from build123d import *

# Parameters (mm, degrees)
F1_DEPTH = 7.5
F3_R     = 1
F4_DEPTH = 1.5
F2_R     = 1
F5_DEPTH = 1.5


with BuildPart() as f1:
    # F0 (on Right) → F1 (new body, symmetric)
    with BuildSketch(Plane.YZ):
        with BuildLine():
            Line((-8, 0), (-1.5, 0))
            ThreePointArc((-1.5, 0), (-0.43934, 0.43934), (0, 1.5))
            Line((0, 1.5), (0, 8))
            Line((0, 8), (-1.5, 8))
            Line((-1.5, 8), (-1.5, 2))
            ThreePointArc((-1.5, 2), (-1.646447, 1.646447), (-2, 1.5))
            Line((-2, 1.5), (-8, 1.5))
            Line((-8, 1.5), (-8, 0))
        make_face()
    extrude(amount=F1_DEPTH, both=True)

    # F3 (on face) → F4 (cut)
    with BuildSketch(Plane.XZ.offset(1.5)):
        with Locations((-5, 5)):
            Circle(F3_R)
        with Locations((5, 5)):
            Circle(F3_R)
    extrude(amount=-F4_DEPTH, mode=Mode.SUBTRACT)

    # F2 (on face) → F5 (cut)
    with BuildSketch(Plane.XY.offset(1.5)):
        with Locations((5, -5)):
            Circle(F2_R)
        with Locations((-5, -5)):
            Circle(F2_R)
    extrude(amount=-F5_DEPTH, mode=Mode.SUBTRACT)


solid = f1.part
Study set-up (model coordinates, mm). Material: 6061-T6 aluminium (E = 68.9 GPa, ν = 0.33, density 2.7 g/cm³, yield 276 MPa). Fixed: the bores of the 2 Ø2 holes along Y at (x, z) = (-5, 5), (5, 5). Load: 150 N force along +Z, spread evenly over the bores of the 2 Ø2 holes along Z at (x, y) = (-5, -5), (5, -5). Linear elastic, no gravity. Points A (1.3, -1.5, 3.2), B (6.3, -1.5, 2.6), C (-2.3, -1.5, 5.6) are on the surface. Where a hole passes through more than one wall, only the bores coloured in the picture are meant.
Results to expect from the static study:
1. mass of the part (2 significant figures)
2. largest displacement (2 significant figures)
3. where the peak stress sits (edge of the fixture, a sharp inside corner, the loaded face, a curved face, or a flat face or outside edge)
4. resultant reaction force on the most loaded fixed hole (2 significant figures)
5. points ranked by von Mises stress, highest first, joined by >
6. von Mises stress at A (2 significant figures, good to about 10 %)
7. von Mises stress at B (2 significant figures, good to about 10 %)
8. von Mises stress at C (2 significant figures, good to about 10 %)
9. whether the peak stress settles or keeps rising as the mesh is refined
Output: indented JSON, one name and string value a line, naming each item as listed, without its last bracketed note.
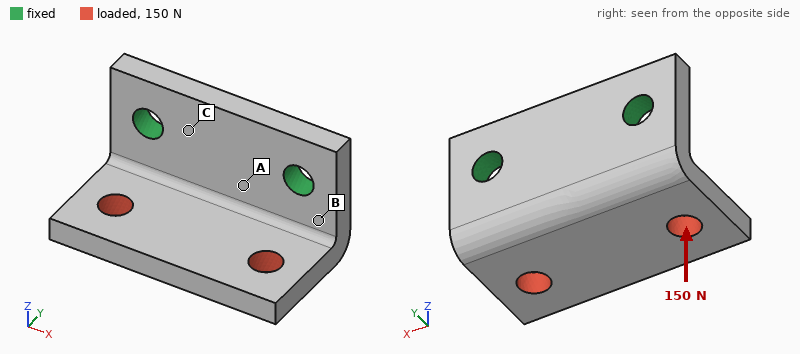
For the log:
{
  "mass of the part": "0.81 g",
  "largest displacement": "82 µm",
  "where the peak stress sits": "edge of the fixture",
  "resultant reaction force on the most loaded fixed hole": "76 N",
  "points ranked by von Mises stress, highest first, joined by >": "B > A > C",
  "von Mises stress at A": "78 MPa",
  "von Mises stress at B": "120 MPa",
  "von Mises stress at C": "32 MPa",
  "whether the peak stress settles or keeps rising as the mesh is refined": "keeps rising"
}
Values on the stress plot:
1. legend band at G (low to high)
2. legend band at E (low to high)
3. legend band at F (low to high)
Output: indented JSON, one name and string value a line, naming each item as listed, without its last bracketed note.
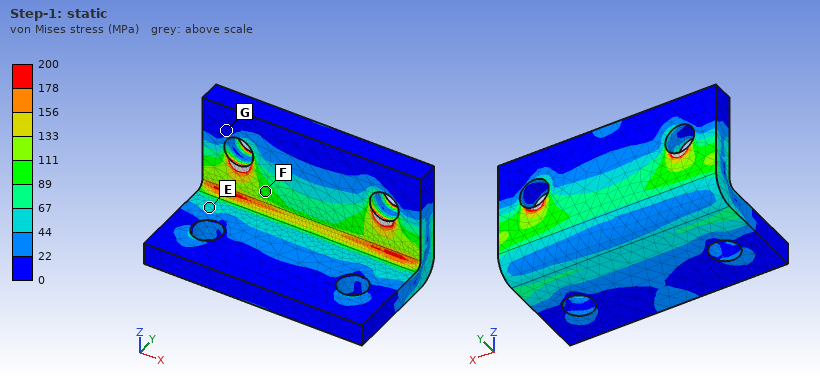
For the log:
{
  "legend band at G": "0 to 22 MPa",
  "legend band at E": "44 to 67 MPa",
  "legend band at F": "89 to 111 MPa"
}
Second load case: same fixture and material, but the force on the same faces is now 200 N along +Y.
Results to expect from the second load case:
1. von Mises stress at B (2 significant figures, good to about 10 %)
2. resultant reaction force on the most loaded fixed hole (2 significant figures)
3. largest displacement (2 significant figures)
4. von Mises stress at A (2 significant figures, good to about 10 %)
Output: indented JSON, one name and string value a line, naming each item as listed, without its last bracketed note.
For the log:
{
  "von Mises stress at B": "73 MPa",
  "resultant reaction force on the most loaded fixed hole": "100 N",
  "largest displacement": "44 µm",
  "von Mises stress at A": "47 MPa"
}
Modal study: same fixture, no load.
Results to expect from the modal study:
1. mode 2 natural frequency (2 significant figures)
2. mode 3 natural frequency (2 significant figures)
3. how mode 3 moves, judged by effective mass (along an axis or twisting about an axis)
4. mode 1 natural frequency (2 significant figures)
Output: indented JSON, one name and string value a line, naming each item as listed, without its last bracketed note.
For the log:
{
  "mode 2 natural frequency": "23 kHz",
  "mode 3 natural frequency": "38 kHz",
  "how mode 3 moves, judged by effective mass": "along X",
  "mode 1 natural frequency": "13 kHz"
}
